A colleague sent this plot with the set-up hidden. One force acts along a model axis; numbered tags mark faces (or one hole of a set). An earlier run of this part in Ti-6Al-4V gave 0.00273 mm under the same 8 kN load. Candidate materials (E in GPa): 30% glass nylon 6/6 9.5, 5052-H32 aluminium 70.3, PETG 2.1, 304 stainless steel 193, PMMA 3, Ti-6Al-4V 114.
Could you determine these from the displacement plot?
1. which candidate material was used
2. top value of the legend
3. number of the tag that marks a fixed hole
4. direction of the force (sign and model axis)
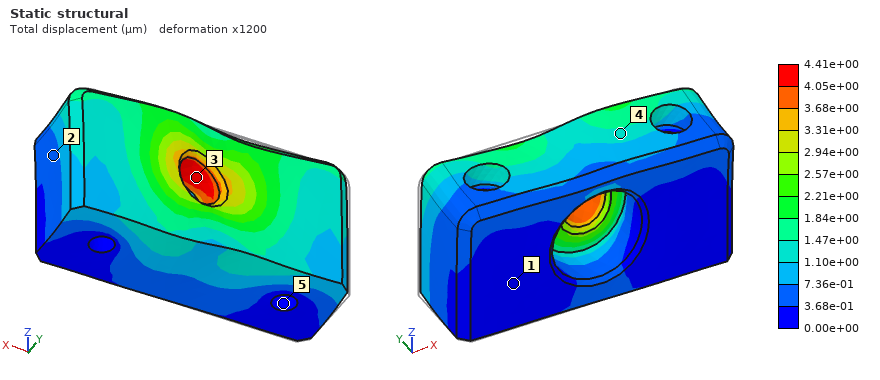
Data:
5052-H32 aluminium
4.41e+00 µm
5
+X
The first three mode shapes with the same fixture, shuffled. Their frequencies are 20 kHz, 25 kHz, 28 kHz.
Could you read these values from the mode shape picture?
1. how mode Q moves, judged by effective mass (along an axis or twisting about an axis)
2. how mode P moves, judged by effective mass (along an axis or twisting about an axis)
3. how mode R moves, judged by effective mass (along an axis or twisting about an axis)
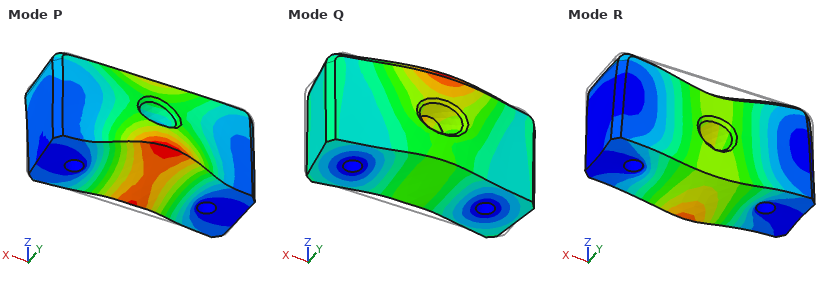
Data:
along Y
twisting about X
along Z
